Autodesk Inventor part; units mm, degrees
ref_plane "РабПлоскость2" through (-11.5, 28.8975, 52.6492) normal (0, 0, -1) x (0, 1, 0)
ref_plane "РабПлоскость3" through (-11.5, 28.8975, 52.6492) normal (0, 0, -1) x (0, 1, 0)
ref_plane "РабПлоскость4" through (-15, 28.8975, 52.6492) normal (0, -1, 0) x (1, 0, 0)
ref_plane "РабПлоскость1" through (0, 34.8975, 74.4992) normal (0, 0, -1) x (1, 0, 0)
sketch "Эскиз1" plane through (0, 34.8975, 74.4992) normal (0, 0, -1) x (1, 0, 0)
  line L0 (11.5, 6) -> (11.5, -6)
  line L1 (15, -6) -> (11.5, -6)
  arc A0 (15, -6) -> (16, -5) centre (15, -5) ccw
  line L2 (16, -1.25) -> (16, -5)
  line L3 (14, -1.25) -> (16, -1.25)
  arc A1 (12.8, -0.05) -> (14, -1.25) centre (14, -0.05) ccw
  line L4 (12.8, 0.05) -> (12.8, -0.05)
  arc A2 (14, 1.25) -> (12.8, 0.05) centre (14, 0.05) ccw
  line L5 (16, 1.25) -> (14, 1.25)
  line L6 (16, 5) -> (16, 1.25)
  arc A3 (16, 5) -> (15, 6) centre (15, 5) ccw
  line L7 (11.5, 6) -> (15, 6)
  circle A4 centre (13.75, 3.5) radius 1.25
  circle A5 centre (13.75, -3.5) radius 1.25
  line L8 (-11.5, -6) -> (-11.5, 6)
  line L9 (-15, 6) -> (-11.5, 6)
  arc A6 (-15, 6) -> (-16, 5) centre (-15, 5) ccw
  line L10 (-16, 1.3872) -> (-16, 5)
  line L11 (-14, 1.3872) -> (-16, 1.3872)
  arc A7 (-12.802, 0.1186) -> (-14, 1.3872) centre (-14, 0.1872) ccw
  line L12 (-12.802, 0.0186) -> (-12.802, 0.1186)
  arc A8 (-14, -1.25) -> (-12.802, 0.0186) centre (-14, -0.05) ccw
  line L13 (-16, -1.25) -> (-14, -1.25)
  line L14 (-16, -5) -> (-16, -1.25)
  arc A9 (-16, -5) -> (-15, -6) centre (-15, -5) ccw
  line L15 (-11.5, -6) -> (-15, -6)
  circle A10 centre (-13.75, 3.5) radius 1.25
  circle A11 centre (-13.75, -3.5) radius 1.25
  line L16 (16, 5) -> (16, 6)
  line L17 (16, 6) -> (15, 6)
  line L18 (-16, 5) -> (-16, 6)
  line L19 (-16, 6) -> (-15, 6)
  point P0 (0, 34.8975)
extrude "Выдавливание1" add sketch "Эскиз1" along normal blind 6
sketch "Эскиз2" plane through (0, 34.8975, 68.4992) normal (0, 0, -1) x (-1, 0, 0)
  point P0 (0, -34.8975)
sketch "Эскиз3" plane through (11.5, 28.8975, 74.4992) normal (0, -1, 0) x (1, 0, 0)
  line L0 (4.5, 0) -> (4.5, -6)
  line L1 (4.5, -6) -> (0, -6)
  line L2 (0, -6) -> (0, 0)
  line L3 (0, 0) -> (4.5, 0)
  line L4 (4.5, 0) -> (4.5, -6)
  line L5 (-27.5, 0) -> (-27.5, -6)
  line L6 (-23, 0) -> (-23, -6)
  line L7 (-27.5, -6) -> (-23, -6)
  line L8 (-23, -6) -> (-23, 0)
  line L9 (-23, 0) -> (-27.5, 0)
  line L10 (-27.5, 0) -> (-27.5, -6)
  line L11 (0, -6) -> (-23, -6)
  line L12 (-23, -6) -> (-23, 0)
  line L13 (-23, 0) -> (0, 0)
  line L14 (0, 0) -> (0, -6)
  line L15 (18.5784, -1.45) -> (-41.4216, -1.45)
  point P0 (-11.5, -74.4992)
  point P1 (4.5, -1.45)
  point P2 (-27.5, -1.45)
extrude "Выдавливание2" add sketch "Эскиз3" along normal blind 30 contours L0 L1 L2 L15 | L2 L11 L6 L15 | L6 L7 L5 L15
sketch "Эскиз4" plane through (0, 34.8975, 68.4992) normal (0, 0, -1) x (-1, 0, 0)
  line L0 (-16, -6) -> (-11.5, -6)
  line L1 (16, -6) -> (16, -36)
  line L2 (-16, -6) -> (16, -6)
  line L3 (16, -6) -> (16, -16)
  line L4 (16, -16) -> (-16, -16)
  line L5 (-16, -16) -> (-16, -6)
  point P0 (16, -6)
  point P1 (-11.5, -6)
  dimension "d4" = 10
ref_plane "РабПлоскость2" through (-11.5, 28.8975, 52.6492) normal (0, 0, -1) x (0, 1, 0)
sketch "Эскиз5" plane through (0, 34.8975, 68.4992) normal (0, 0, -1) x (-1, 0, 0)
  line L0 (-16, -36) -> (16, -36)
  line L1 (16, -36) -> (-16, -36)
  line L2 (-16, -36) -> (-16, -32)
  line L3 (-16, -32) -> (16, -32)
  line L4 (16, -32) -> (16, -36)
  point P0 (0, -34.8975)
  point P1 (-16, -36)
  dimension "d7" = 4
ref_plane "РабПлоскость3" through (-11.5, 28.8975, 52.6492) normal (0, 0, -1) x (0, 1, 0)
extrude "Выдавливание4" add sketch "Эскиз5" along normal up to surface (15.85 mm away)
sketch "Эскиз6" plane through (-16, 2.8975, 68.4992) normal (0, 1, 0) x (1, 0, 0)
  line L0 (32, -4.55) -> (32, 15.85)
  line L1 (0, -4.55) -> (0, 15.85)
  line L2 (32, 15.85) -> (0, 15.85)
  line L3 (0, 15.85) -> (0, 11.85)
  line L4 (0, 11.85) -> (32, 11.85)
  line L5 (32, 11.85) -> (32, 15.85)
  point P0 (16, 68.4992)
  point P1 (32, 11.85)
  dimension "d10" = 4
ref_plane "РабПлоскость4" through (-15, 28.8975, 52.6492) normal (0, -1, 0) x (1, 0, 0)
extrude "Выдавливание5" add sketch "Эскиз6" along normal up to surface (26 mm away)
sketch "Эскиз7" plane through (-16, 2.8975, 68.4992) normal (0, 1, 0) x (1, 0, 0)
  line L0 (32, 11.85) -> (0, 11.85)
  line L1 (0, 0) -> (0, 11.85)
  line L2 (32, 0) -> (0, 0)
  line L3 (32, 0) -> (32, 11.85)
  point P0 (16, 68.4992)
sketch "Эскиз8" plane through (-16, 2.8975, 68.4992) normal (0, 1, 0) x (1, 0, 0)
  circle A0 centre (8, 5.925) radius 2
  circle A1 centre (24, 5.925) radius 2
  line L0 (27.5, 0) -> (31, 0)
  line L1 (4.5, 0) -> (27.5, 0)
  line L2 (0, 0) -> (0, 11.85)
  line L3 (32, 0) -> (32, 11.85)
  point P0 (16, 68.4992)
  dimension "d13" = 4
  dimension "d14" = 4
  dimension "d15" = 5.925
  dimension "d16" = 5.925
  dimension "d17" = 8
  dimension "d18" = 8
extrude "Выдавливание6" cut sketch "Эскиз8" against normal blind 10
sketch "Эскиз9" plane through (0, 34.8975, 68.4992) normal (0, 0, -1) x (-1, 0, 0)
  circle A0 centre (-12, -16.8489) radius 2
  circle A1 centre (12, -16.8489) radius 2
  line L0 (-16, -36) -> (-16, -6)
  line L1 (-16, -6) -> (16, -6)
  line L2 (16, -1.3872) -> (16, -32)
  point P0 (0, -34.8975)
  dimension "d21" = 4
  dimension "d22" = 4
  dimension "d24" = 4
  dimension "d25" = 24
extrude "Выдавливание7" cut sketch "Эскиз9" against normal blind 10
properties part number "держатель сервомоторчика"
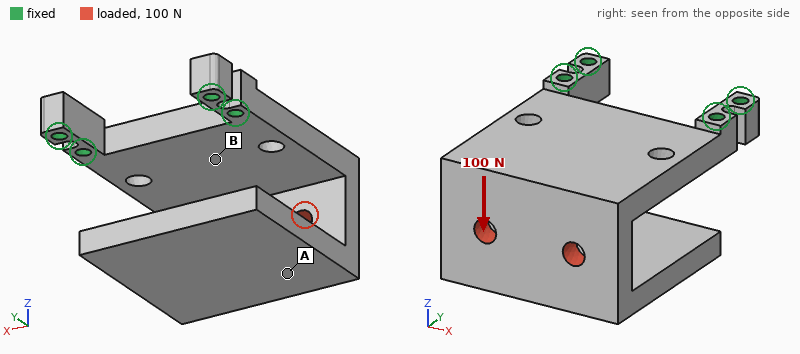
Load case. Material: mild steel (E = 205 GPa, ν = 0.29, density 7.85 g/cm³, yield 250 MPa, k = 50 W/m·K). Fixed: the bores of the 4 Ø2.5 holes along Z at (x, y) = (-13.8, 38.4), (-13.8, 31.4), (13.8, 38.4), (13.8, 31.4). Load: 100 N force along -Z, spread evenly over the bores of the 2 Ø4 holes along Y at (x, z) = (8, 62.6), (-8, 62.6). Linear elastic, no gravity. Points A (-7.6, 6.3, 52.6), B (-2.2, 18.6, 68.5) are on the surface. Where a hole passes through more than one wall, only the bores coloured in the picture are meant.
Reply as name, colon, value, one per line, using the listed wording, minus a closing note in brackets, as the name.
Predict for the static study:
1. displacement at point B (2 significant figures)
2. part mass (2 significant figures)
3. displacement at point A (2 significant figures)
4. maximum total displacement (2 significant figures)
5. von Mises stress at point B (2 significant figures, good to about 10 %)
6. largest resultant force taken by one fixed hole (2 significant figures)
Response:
displacement at point B: 11 µm
part mass: 78 g
displacement at point A: 40 µm
maximum total displacement: 49 µm
von Mises stress at point B: 15 MPa
largest resultant force taken by one fixed hole: 53 N
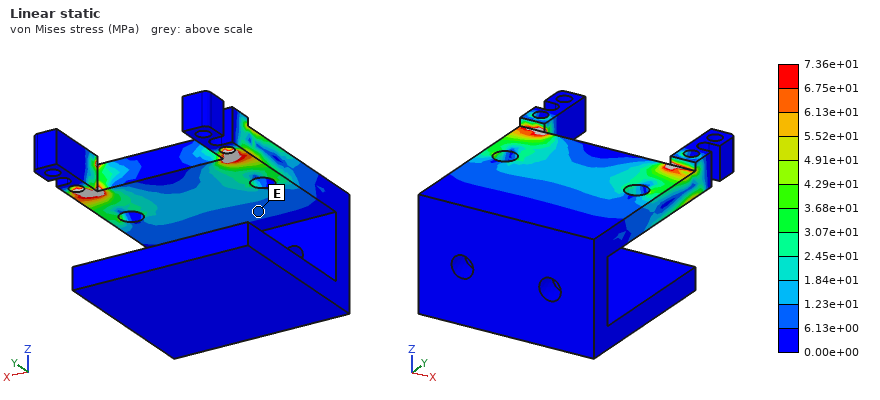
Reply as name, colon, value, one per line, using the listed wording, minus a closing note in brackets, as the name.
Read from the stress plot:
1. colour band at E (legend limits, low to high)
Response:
colour band at E: 6.13e+00 to 1.23e+01 MPa
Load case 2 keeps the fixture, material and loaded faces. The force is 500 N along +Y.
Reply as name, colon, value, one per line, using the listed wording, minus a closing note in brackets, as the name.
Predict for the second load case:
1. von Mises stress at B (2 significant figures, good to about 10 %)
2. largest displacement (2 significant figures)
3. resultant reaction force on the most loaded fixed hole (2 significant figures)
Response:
von Mises stress at B: 36 MPa
largest displacement: 0.10 mm
resultant reaction force on the most loaded fixed hole: 260 N
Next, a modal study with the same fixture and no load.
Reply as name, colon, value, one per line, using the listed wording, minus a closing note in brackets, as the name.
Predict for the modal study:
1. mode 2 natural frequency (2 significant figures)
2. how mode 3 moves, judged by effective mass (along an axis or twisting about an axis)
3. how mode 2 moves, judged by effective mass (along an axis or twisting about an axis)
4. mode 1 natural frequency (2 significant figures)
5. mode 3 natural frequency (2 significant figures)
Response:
mode 2 natural frequency: 1900 Hz
how mode 3 moves, judged by effective mass: along X
how mode 2 moves, judged by effective mass: along Z
mode 1 natural frequency: 1200 Hz
mode 3 natural frequency: 2100 Hz
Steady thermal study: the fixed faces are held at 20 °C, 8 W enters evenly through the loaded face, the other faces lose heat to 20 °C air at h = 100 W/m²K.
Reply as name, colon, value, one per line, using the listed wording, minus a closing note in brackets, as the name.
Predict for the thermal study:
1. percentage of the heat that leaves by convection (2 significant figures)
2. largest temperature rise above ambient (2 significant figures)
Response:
percentage of the heat that leaves by convection: 77 %
largest temperature rise above ambient: 20 K
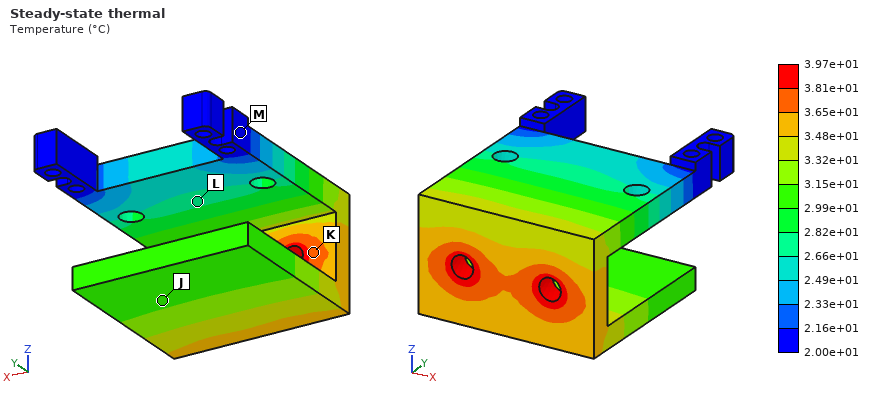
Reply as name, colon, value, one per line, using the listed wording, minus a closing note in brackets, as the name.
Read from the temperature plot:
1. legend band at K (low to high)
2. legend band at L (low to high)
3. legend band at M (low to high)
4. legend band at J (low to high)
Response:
legend band at K: 3.65e+01 to 3.81e+01 °C
legend band at L: 2.66e+01 to 2.82e+01 °C
legend band at M: 2.00e+01 to 2.16e+01 °C
legend band at J: 2.99e+01 to 3.15e+01 °C
